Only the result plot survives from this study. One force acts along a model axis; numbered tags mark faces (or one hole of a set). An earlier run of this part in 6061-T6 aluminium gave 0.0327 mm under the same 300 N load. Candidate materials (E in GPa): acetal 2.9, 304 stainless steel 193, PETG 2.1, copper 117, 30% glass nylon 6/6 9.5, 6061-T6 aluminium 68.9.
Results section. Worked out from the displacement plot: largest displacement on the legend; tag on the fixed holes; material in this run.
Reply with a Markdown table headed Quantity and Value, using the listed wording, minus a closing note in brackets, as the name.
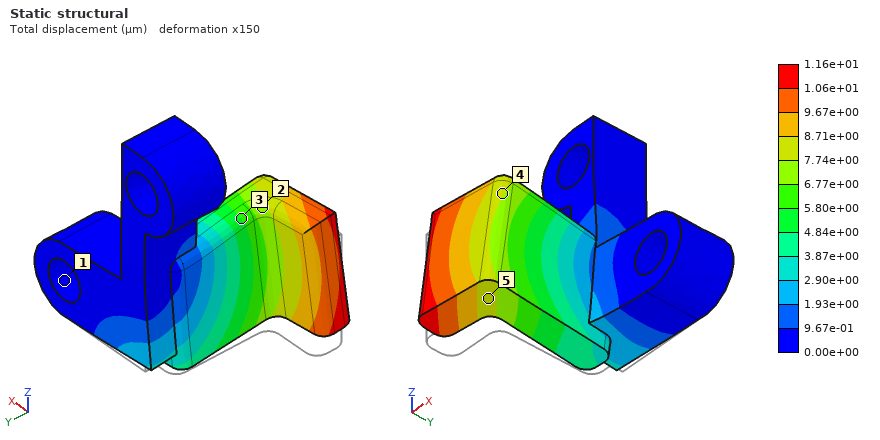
| Quantity | Value |
|---|---|
| largest displacement on the legend | 1.16e+01 µm |
| tag on the fixed holes | 1 |
| material in this run | 304 stainless steel |
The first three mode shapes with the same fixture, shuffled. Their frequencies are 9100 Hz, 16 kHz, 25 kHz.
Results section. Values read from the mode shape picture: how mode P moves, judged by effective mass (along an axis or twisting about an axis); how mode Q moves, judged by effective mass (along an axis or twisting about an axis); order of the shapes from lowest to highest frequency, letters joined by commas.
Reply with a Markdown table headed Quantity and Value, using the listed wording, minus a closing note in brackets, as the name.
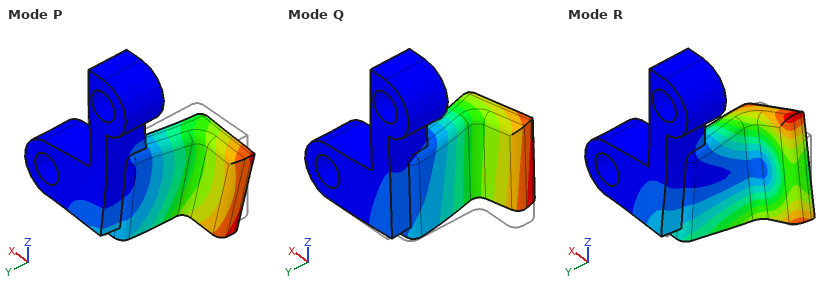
| Quantity | Value |
|---|---|
| how mode P moves, judged by effective mass | along Z |
| how mode Q moves, judged by effective mass | along X |
| order of the shapes from lowest to highest frequency, letters joined by commas | Q, P, R |
